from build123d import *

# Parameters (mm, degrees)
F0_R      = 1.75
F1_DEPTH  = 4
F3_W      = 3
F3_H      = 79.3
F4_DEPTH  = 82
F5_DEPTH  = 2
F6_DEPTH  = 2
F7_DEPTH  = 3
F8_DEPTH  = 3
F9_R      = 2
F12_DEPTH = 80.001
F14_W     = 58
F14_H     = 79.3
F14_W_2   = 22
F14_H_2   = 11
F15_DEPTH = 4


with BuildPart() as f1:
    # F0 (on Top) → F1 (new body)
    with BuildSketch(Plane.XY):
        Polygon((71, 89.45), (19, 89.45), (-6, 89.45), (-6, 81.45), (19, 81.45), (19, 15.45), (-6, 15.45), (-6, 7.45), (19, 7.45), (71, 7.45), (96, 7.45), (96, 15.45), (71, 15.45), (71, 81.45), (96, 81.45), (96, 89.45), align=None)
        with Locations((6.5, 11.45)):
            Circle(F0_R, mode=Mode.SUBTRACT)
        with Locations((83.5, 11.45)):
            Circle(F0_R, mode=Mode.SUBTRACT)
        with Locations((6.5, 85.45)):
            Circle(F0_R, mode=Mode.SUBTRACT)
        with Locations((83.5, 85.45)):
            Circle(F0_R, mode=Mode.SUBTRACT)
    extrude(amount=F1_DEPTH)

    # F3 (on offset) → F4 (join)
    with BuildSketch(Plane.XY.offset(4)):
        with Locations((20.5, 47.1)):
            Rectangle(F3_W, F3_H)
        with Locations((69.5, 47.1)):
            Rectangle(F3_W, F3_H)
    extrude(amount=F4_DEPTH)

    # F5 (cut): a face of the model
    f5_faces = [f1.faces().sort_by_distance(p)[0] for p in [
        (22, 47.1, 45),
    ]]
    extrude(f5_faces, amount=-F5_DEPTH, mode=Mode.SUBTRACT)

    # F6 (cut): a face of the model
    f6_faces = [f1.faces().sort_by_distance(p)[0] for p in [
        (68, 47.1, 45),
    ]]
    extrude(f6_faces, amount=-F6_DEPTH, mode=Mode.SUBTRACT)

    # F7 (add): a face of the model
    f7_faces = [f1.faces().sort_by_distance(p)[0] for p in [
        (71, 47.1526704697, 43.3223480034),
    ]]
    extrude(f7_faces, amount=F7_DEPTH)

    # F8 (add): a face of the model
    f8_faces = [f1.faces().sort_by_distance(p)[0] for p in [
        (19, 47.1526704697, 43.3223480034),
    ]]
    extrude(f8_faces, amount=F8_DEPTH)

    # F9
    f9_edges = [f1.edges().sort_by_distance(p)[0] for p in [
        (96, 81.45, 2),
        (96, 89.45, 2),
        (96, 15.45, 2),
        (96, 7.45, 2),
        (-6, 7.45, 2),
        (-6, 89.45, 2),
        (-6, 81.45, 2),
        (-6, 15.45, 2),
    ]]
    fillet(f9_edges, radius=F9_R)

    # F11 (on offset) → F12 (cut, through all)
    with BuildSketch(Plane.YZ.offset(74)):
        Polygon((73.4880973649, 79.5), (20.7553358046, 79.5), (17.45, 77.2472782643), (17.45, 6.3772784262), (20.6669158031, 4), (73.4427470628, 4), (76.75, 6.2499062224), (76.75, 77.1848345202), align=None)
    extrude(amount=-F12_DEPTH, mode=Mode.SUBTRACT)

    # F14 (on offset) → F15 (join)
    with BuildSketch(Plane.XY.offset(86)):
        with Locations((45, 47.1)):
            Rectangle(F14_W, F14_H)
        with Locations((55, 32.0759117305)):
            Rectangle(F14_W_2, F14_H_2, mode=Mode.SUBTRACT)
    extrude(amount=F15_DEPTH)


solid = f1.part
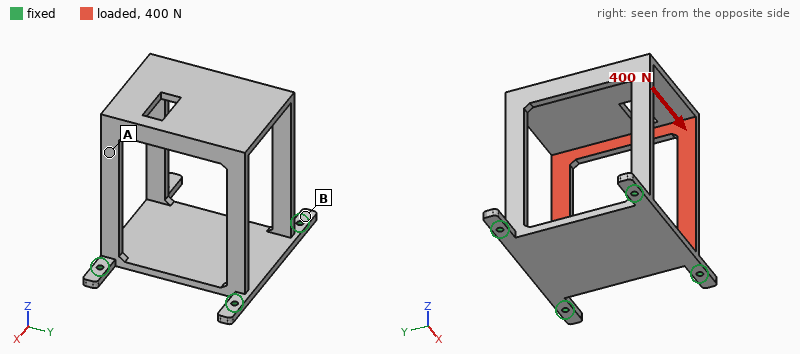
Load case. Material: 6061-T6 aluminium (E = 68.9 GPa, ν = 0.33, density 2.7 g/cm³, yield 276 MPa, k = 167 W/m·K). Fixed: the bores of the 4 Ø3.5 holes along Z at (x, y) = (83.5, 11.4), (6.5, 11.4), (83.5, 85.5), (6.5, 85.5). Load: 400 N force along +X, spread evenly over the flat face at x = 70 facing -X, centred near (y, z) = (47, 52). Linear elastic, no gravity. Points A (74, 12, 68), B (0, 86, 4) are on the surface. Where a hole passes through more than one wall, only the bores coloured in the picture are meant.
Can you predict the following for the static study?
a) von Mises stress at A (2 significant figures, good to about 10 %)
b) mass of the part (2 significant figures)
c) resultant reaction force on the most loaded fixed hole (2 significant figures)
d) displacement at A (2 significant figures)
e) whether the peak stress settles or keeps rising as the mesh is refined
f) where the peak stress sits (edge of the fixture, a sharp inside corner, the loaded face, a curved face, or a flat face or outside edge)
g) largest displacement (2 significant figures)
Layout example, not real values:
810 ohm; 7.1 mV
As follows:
57 MPa; 150 g; 190 N; 0.80 mm; keeps rising; a sharp inside corner; 0.88 mm
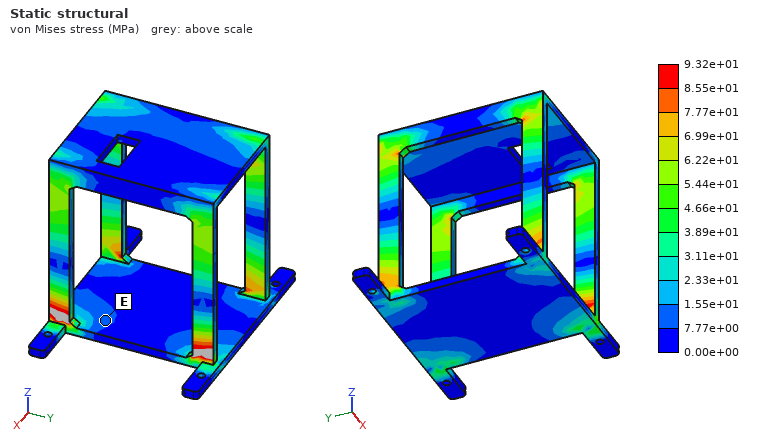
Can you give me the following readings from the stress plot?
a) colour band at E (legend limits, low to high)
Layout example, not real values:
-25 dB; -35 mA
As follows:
7.77e+00 to 1.55e+01 MPa
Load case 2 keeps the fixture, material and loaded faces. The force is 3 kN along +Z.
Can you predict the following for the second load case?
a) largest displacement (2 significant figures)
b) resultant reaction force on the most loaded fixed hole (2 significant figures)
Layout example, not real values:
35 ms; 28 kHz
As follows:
0.29 mm; 1.4 kN
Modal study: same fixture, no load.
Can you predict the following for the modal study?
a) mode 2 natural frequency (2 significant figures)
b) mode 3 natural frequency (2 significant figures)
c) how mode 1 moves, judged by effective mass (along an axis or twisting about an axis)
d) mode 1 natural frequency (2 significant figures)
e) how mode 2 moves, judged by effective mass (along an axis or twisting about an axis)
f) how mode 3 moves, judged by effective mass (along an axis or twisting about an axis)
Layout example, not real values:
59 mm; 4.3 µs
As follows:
630 Hz; 680 Hz; along X; 320 Hz; along Y; twisting about Z
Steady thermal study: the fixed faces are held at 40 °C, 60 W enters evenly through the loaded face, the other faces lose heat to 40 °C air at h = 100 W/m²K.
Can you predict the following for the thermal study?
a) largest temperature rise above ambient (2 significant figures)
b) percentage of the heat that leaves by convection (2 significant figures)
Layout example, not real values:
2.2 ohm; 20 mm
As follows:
50 K; 74 %
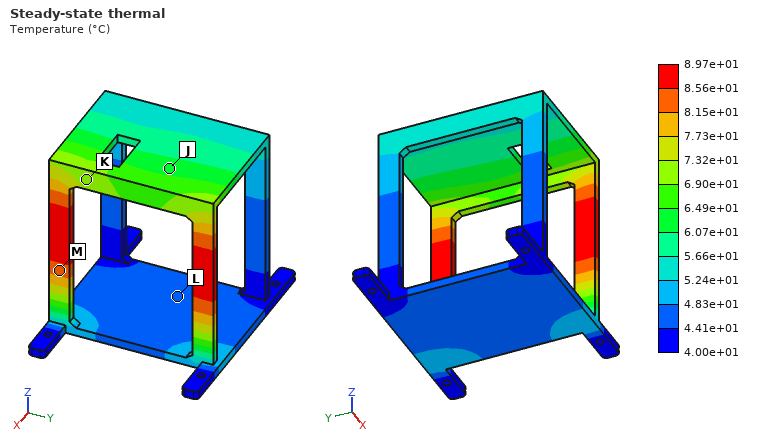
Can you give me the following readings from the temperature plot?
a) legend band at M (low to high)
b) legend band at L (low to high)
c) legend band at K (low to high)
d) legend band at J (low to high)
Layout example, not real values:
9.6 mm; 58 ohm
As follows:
8.15e+01 to 8.56e+01 °C; 4.41e+01 to 4.83e+01 °C; 6.90e+01 to 7.32e+01 °C; 6.07e+01 to 6.49e+01 °C
